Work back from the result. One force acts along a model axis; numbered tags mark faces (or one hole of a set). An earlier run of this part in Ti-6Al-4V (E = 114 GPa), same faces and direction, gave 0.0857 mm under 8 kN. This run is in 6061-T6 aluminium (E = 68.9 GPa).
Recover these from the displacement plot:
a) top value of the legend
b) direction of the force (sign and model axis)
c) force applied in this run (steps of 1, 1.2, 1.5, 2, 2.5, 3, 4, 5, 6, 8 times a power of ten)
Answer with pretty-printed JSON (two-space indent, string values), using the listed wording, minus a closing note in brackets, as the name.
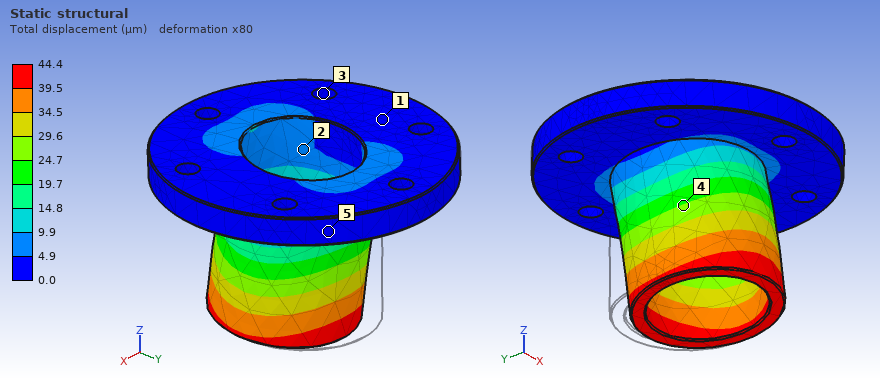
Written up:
{
  "top value of the legend": "44.4 µm",
  "direction of the force": "-Y",
  "force applied in this run": "2.5 kN"
}
